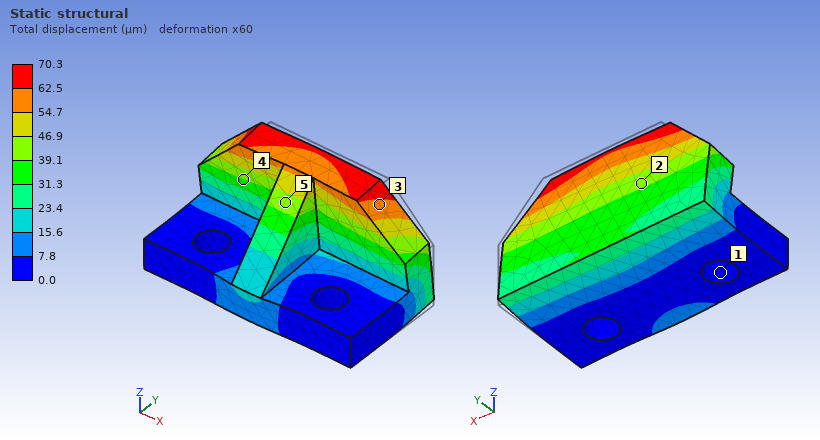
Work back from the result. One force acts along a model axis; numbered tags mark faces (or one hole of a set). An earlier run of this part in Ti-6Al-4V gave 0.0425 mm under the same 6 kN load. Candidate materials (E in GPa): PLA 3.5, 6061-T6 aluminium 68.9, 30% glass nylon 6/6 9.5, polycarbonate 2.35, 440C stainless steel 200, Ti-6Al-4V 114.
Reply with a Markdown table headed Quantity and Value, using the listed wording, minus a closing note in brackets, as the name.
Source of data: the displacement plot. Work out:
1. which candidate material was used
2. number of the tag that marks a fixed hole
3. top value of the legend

| Quantity | Value |
|---|---|
| which candidate material was used | 6061-T6 aluminium |
| number of the tag that marks a fixed hole | 1 |
| top value of the legend | 70.3 µm |
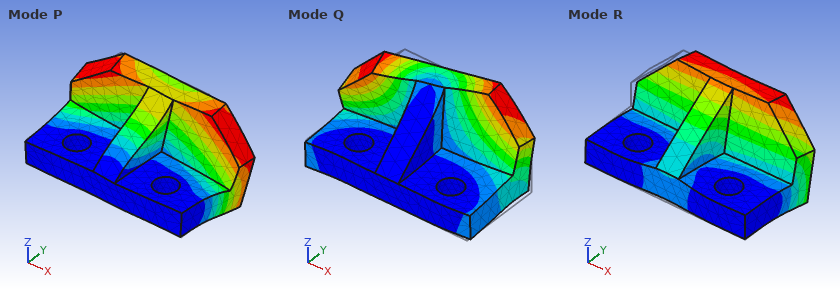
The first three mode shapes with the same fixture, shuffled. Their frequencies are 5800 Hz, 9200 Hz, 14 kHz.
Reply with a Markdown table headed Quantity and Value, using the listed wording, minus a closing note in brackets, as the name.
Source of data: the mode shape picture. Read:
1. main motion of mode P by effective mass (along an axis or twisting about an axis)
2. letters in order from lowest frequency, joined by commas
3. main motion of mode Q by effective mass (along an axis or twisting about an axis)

| Quantity | Value |
|---|---|
| main motion of mode P by effective mass | along X |
| letters in order from lowest frequency, joined by commas | R, P, Q |
| main motion of mode Q by effective mass | along X |
